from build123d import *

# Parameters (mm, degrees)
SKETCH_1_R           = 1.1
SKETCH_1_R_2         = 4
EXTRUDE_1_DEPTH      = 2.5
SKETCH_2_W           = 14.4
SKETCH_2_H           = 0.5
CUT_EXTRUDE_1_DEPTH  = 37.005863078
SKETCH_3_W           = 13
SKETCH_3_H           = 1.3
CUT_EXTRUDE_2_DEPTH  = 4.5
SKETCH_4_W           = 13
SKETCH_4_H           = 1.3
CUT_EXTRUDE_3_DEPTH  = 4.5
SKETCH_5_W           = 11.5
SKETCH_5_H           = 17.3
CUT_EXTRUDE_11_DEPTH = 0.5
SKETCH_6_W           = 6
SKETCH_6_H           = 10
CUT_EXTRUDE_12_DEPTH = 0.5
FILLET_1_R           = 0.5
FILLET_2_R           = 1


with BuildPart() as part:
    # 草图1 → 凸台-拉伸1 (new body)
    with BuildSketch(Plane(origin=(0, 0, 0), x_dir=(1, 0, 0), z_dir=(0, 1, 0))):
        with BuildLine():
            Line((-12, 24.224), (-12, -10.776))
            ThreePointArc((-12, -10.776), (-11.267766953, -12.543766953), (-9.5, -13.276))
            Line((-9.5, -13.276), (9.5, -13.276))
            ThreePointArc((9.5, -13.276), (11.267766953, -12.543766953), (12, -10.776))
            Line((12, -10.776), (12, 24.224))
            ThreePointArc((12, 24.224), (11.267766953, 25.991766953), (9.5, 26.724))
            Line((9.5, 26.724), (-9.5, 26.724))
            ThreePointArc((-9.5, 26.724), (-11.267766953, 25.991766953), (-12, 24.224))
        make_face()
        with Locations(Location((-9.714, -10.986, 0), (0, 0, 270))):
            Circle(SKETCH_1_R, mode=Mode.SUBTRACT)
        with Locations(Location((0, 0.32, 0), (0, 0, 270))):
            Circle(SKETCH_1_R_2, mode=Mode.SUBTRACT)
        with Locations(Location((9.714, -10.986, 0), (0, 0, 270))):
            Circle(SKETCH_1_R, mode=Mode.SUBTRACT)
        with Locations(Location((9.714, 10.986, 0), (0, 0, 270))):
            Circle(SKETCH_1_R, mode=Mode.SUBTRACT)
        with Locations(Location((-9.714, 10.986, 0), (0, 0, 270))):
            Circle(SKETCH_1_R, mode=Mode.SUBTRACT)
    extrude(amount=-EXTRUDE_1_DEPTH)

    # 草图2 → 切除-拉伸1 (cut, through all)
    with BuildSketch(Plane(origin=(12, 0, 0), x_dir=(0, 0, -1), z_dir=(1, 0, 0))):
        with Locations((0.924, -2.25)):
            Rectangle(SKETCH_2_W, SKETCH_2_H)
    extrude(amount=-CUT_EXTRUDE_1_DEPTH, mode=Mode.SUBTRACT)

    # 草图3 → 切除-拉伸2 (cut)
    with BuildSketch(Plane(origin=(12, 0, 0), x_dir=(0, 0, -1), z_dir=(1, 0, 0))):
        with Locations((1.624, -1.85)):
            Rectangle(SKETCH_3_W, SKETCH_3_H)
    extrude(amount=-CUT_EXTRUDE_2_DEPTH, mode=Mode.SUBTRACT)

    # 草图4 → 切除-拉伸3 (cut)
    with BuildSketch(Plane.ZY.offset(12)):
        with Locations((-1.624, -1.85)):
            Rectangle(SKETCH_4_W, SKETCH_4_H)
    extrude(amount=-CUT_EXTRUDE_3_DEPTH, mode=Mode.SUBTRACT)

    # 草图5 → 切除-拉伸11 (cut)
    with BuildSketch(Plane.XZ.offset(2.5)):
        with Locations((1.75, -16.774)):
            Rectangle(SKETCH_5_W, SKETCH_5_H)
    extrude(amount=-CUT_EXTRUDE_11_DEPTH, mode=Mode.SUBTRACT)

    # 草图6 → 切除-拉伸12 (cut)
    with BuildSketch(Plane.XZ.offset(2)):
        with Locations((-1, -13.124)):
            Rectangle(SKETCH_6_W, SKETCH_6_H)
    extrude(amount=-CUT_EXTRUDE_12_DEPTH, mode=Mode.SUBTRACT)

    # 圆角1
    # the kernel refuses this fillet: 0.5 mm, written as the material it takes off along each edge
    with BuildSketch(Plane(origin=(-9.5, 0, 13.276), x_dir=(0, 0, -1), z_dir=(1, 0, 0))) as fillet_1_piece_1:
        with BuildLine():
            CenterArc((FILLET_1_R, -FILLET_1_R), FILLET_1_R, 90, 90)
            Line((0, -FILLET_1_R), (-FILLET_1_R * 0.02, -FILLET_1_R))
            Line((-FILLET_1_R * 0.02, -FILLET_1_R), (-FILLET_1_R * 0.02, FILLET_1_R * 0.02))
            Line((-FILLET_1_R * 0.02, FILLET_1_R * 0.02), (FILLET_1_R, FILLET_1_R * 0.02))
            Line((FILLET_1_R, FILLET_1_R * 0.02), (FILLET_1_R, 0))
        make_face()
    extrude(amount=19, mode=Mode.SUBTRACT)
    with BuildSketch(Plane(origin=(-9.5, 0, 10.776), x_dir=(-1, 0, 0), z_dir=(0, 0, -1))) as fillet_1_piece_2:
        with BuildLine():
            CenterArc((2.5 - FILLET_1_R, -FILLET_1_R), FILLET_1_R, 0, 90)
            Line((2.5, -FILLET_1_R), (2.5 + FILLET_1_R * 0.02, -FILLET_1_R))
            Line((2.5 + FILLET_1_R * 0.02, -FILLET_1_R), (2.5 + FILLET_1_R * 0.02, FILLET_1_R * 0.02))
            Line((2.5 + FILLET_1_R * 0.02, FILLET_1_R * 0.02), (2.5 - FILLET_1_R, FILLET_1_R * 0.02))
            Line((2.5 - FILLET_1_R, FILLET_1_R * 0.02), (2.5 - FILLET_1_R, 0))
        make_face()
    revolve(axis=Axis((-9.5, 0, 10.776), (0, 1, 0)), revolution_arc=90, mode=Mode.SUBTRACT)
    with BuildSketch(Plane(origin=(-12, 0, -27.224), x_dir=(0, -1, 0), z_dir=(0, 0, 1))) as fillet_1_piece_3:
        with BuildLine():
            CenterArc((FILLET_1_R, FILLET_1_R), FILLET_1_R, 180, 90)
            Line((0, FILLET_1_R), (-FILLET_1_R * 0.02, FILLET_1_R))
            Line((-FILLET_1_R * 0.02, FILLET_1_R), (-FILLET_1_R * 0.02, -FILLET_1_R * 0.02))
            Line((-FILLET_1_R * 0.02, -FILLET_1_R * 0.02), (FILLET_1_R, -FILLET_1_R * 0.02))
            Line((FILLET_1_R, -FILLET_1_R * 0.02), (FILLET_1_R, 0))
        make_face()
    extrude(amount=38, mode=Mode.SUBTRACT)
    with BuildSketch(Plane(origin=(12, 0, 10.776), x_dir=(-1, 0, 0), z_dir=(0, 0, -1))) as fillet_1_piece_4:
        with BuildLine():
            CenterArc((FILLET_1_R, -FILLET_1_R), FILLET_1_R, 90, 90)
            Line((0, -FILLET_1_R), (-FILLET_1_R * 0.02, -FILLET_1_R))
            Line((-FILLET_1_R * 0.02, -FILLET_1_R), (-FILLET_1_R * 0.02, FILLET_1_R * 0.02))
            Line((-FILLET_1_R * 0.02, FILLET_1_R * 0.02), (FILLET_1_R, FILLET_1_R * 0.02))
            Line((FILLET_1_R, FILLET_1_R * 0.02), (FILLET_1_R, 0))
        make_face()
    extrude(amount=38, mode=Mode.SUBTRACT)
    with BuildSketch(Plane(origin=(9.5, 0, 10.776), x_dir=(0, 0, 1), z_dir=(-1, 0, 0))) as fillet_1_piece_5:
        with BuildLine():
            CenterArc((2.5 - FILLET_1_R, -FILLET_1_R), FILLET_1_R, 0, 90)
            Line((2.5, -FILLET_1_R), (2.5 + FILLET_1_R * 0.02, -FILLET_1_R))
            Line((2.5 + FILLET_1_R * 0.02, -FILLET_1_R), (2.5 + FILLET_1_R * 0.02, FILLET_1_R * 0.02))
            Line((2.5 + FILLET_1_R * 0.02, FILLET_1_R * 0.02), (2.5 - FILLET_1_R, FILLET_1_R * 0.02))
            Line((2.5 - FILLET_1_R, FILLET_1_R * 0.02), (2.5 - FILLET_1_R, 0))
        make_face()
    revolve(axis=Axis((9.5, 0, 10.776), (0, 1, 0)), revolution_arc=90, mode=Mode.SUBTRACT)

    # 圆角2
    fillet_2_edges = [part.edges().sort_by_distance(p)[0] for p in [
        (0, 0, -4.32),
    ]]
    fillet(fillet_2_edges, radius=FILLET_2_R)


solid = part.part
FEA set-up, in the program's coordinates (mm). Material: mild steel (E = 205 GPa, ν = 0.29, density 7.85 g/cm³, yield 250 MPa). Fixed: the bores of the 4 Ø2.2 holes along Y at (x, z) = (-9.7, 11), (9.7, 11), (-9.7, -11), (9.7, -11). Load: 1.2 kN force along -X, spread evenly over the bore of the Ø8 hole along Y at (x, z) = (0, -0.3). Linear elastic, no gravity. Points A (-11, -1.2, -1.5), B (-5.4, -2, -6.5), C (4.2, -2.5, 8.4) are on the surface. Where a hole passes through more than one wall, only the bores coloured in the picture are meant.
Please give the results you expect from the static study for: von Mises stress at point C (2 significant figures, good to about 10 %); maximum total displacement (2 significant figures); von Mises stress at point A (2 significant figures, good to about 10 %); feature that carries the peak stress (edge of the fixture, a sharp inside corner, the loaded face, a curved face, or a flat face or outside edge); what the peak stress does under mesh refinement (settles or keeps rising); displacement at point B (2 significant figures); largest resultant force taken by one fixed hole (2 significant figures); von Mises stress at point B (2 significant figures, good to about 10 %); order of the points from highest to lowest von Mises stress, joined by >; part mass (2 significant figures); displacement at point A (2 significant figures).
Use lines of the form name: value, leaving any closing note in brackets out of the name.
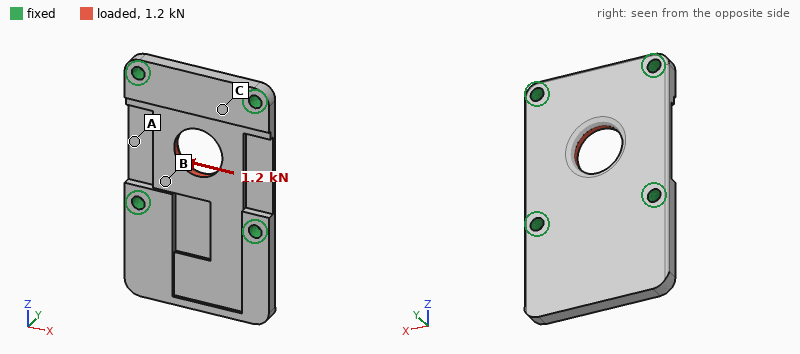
von Mises stress at point C: 23 MPa
maximum total displacement: 2.9 µm
von Mises stress at point A: 9.9 MPa
feature that carries the peak stress: edge of the fixture
what the peak stress does under mesh refinement: keeps rising
displacement at point B: 1.2 µm
largest resultant force taken by one fixed hole: 350 N
von Mises stress at point B: 37 MPa
order of the points from highest to lowest von Mises stress, joined by >: B > C > A
part mass: 14 g
displacement at point A: 2.3 µm
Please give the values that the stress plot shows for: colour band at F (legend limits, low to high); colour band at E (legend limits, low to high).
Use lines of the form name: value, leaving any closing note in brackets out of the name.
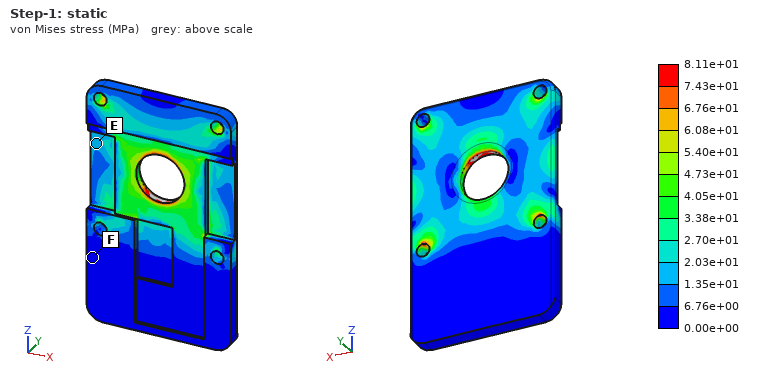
colour band at F: 0.00e+00 to 6.76e+00 MPa
colour band at E: 1.35e+01 to 2.03e+01 MPa
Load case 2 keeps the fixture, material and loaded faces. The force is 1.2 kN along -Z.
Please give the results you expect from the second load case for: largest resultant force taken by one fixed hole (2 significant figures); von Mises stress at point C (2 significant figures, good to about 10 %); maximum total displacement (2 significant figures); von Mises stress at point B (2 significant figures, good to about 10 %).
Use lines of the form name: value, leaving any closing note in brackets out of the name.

largest resultant force taken by one fixed hole: 330 N
von Mises stress at point C: 17 MPa
maximum total displacement: 2.1 µm
von Mises stress at point B: 34 MPa
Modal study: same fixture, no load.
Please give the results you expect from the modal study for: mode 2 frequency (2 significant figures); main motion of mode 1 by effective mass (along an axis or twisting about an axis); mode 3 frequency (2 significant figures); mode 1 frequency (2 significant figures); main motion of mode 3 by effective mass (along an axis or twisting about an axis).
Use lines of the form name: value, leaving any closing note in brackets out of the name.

mode 2 frequency: 14 kHz
main motion of mode 1 by effective mass: along Y
mode 3 frequency: 20 kHz
mode 1 frequency: 7100 Hz
main motion of mode 3 by effective mass: along Y
